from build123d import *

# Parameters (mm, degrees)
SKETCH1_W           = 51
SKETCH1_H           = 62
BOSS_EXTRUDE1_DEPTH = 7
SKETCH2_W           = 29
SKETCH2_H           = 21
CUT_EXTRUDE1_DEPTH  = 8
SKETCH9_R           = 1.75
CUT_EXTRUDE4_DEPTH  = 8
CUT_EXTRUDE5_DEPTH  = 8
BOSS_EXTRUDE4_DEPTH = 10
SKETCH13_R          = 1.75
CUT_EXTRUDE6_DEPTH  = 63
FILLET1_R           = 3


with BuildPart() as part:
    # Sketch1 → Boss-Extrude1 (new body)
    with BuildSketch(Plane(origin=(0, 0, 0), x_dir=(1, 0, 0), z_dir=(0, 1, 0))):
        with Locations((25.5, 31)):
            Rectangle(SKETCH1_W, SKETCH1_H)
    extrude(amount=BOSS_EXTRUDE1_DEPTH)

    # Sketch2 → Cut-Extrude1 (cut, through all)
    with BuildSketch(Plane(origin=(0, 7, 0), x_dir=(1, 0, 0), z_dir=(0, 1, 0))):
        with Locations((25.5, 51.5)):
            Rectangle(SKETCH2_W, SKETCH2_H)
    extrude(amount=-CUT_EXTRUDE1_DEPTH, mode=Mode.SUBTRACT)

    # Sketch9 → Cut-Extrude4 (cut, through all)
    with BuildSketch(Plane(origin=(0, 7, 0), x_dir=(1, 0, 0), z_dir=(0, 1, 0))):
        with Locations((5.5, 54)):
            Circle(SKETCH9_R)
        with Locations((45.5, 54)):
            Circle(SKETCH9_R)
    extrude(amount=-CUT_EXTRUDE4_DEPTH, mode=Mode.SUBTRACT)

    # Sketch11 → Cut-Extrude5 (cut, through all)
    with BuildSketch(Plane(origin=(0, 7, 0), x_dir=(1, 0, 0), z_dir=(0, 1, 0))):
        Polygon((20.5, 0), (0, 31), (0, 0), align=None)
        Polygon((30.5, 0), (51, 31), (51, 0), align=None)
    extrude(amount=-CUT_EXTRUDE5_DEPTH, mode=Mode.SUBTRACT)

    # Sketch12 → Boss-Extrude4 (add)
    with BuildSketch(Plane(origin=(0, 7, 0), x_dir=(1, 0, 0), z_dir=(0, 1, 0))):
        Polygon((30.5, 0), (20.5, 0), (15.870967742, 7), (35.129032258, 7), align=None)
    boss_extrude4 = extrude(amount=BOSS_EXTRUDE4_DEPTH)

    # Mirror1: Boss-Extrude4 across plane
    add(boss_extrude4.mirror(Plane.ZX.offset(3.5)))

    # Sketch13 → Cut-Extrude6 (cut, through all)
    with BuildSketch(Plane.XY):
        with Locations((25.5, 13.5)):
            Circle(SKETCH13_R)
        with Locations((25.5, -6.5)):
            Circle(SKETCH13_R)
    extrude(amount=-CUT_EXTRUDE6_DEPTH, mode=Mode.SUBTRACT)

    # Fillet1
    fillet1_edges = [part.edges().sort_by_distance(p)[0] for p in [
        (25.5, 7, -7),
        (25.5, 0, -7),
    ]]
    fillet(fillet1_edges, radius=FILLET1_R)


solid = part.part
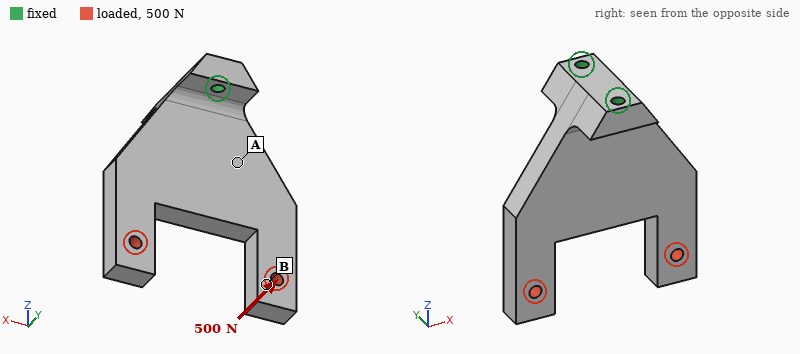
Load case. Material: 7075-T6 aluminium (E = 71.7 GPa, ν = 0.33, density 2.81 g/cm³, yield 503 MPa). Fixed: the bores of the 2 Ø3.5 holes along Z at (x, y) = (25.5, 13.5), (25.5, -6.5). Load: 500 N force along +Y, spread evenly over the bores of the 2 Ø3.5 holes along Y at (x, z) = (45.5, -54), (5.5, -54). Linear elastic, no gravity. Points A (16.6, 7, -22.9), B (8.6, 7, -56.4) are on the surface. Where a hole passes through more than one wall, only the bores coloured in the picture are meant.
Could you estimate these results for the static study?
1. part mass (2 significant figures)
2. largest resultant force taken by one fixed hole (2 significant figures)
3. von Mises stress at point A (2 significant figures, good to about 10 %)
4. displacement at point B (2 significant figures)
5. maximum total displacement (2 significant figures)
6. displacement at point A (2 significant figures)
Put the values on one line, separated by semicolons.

43 g; 1.5 kN; 50 MPa; 0.40 mm; 0.46 mm; 0.079 mm
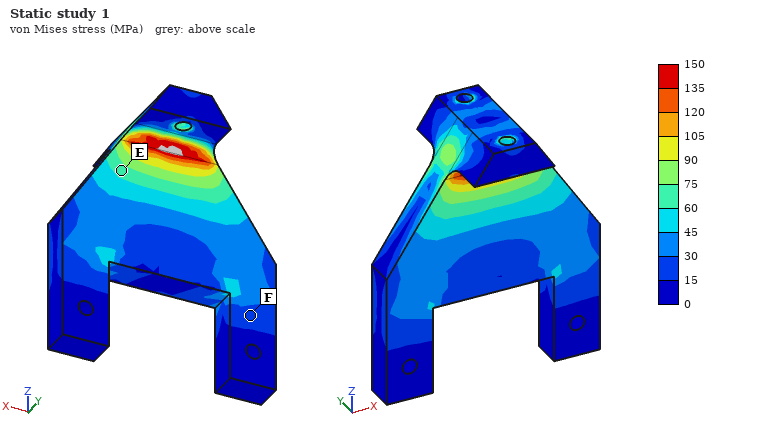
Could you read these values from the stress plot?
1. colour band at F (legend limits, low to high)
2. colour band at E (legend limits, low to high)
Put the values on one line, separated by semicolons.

15 to 30 MPa; 60 to 75 MPa
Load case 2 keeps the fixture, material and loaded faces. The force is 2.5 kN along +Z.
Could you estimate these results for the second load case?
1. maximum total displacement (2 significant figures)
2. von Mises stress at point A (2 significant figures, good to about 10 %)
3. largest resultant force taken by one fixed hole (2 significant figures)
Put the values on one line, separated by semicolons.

25 µm; 11 MPa; 1.3 kN
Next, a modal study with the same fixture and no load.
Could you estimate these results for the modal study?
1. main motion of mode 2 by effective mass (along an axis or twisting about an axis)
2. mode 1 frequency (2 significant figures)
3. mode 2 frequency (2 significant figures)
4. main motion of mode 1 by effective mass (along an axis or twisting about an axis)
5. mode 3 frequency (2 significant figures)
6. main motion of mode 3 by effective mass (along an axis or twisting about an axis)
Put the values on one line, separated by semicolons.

along X; 1700 Hz; 2000 Hz; along Y; 2900 Hz; twisting about Z
